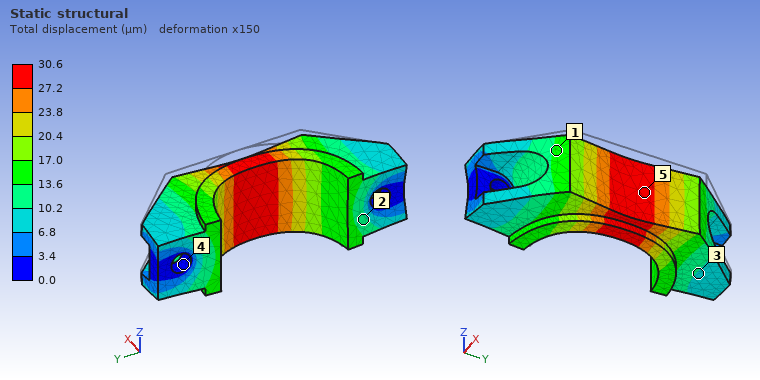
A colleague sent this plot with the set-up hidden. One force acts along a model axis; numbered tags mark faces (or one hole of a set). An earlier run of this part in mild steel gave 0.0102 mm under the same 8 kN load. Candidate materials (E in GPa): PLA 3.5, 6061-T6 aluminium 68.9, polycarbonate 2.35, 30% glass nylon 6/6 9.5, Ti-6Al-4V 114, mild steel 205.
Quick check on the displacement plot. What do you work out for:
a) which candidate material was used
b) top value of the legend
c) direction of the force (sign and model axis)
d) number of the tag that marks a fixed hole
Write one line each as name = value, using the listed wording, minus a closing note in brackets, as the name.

which candidate material was used = 6061-T6 aluminium
top value of the legend = 30.6 µm
direction of the force = -X
number of the tag that marks a fixed hole = 4
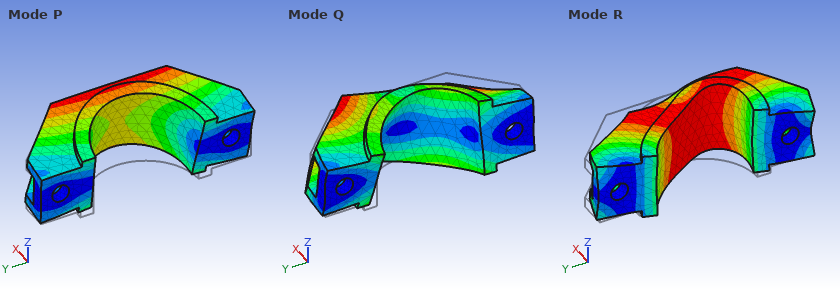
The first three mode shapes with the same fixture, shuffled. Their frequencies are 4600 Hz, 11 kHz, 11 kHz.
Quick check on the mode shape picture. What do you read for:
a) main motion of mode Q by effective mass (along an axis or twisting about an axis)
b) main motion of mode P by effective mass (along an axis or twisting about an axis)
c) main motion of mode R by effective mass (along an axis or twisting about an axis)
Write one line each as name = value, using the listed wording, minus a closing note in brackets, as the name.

main motion of mode Q by effective mass = twisting about X
main motion of mode P by effective mass = along Z
main motion of mode R by effective mass = along Y
